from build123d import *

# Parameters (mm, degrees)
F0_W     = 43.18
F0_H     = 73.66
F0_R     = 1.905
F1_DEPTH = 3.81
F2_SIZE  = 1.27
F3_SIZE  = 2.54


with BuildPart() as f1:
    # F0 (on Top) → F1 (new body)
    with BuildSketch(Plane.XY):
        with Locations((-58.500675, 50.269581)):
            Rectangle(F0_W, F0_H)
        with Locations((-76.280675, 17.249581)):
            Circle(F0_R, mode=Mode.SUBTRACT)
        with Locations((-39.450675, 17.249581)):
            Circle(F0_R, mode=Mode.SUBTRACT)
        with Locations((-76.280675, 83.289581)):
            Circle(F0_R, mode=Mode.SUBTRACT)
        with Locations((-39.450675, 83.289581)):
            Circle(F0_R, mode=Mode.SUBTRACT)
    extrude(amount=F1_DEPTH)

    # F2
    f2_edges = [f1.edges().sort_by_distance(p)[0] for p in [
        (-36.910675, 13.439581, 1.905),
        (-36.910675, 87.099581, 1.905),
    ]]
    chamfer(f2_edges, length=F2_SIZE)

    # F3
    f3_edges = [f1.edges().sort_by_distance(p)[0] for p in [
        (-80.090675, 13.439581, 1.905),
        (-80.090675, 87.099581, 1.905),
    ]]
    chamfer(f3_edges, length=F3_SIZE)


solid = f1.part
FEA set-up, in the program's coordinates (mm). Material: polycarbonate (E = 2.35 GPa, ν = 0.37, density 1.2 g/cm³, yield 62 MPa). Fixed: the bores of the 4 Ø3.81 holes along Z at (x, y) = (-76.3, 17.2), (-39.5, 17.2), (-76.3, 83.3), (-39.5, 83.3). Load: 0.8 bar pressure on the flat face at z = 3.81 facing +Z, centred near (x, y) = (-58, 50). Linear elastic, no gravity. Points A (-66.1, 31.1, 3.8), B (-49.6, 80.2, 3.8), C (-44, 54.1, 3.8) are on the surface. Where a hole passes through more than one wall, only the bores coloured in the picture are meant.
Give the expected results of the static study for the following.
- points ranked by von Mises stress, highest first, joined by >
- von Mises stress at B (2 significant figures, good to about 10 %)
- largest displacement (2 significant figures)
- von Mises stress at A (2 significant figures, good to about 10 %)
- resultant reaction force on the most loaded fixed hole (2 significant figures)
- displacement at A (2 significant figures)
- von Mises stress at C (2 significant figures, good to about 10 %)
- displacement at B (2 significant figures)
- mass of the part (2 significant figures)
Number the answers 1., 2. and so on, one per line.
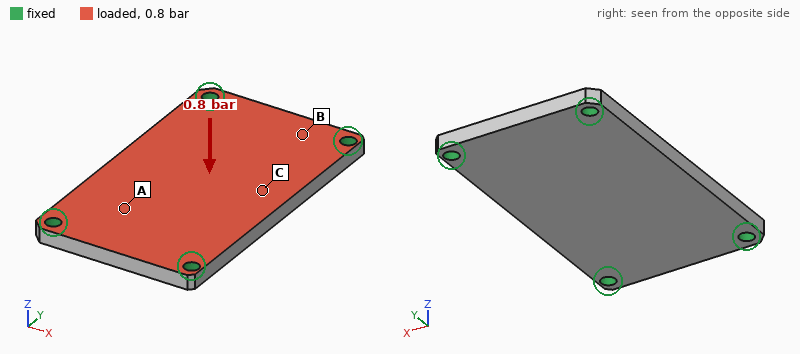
1. C > B > A
2. 3.5 MPa
3. 0.50 mm
4. 2.1 MPa
5. 65 N
6. 0.26 mm
7. 6.5 MPa
8. 0.079 mm
9. 14 g
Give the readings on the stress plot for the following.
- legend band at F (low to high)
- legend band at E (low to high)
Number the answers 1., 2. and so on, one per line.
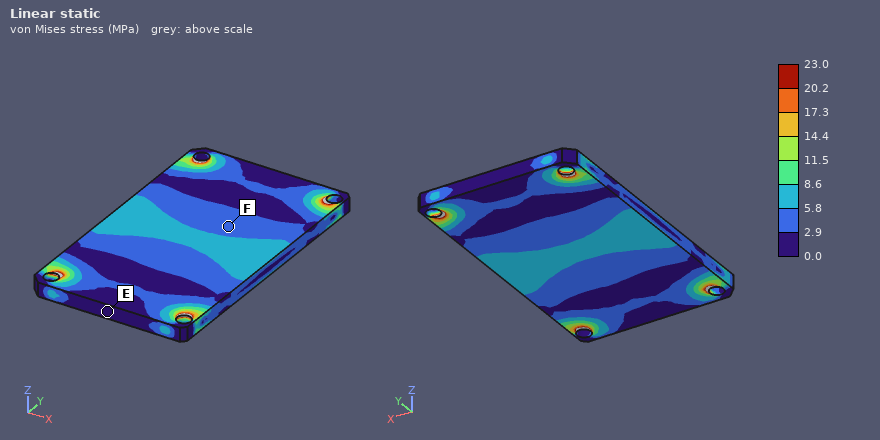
1. 2.9 to 5.8 MPa
2. 0.0 to 2.9 MPa
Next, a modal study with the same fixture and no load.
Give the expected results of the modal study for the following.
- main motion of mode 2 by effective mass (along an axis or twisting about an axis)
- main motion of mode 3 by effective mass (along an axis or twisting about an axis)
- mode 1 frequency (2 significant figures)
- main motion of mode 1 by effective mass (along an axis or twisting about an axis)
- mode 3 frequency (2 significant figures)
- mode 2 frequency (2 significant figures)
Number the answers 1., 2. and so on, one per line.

1. twisting about Y
2. twisting about X
3. 1100 Hz
4. along Z
5. 2900 Hz
6. 1800 Hz
